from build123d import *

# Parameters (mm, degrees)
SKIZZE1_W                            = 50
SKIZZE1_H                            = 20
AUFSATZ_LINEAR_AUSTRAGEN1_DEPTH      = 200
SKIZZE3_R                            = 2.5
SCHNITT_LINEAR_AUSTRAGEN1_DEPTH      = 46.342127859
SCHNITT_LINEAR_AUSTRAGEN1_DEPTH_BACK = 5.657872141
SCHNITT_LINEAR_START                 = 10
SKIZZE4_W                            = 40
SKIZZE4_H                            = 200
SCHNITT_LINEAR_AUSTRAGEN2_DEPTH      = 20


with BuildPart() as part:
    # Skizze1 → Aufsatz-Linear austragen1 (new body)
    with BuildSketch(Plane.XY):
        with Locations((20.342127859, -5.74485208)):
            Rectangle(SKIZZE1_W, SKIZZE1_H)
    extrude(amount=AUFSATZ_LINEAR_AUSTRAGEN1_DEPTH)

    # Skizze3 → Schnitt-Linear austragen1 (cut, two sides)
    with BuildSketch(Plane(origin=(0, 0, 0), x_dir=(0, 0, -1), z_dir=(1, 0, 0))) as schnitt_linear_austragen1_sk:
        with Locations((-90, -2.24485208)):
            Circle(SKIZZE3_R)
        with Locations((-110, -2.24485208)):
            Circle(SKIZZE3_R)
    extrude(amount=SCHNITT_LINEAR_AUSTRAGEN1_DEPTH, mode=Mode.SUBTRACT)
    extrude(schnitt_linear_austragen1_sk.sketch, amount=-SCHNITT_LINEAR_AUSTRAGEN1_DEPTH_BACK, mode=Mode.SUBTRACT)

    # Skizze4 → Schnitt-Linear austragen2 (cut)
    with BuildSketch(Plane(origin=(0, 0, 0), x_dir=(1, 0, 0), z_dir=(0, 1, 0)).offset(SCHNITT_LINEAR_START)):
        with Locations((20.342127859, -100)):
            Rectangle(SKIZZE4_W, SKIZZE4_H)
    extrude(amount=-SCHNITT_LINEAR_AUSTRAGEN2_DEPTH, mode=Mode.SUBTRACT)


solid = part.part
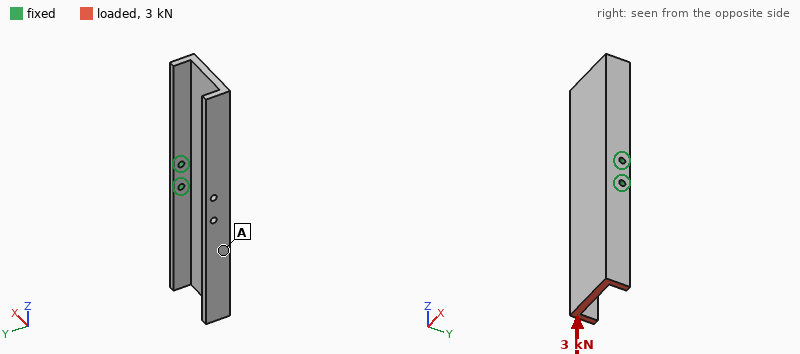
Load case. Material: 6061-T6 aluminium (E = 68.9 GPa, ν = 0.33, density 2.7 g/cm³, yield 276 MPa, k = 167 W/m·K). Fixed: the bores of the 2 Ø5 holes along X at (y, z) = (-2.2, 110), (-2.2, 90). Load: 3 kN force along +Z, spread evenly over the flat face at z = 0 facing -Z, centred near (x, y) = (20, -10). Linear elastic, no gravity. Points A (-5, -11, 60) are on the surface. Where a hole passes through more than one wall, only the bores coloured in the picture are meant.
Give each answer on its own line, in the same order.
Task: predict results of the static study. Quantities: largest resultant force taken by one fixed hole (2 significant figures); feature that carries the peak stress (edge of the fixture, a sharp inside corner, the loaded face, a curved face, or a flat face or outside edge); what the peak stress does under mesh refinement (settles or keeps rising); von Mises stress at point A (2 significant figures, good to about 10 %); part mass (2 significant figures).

3.2 kN
edge of the fixture
keeps rising
14 MPa
230 g
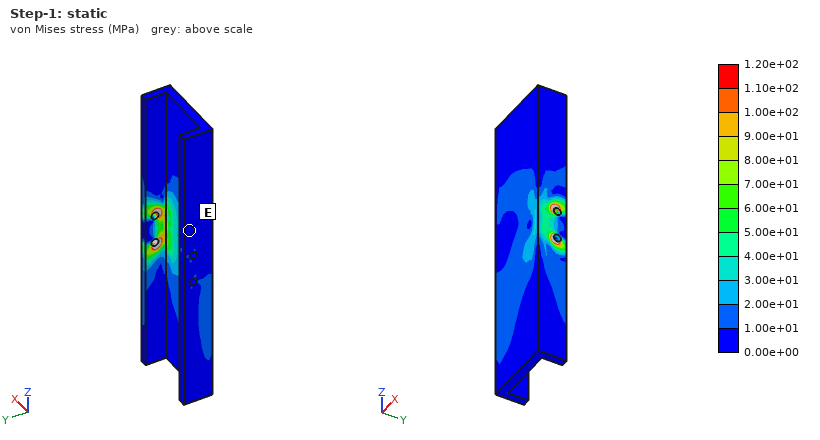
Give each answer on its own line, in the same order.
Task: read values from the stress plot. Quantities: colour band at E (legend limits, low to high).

0.00e+00 to 1.00e+01 MPa
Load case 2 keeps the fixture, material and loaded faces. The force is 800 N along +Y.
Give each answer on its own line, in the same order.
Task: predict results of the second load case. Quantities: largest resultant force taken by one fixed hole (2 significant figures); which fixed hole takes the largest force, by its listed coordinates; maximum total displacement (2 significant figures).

3.5 kN
(-2.2, 90)
1.2 mm
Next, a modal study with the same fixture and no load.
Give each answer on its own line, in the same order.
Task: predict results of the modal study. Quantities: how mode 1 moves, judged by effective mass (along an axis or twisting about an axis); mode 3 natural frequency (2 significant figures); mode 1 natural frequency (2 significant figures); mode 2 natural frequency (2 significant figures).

along Y
820 Hz
600 Hz
630 Hz
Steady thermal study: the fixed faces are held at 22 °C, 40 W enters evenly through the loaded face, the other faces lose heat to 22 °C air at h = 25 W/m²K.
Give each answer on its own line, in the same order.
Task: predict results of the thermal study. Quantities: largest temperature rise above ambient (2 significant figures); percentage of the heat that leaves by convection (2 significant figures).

52 K
36 %
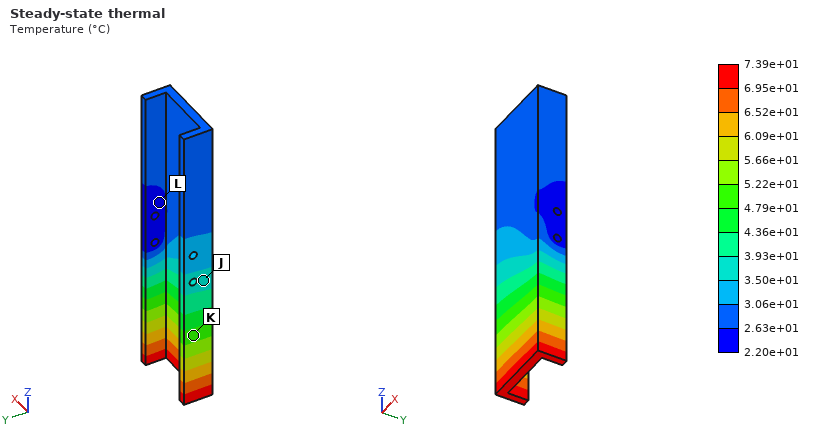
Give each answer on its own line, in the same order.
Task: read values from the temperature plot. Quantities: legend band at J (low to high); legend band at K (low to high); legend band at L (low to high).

3.50e+01 to 3.93e+01 °C
4.79e+01 to 5.22e+01 °C
2.20e+01 to 2.63e+01 °C
